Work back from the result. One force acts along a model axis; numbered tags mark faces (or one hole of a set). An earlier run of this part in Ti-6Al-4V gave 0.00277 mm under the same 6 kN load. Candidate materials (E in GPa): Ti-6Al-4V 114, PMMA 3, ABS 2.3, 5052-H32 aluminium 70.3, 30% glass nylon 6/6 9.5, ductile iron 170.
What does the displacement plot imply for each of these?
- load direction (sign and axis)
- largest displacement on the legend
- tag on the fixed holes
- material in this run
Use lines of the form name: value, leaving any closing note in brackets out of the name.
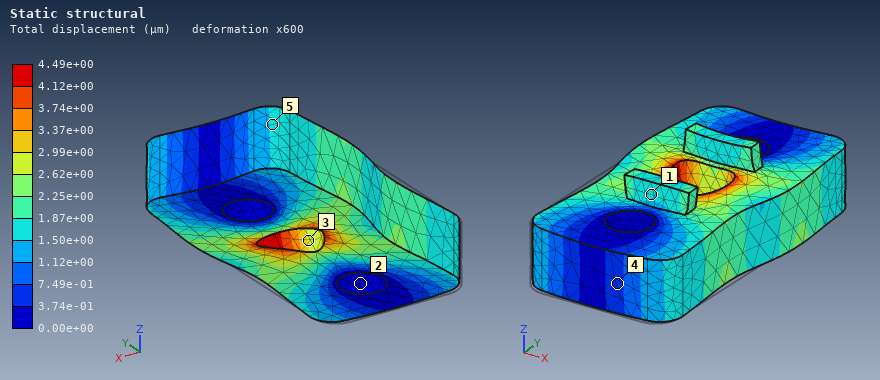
load direction: +Y
largest displacement on the legend: 4.49e+00 µm
tag on the fixed holes: 2
material in this run: 5052-H32 aluminium
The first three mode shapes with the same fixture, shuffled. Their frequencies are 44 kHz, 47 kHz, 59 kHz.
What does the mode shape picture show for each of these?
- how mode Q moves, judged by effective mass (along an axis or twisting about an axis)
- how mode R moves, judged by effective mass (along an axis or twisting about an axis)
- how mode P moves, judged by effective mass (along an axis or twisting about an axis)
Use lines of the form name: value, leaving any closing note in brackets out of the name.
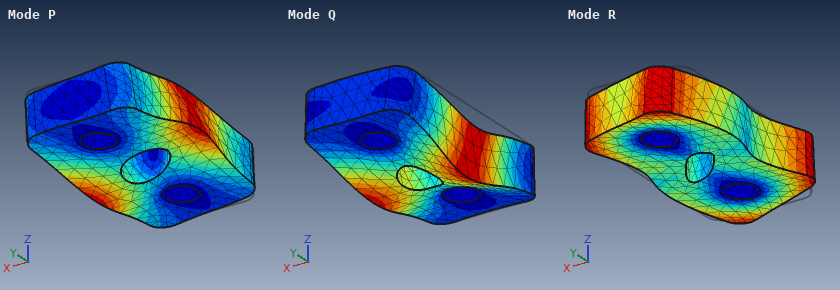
how mode Q moves, judged by effective mass: along Z
how mode R moves, judged by effective mass: twisting about Z
how mode P moves, judged by effective mass: twisting about Y
